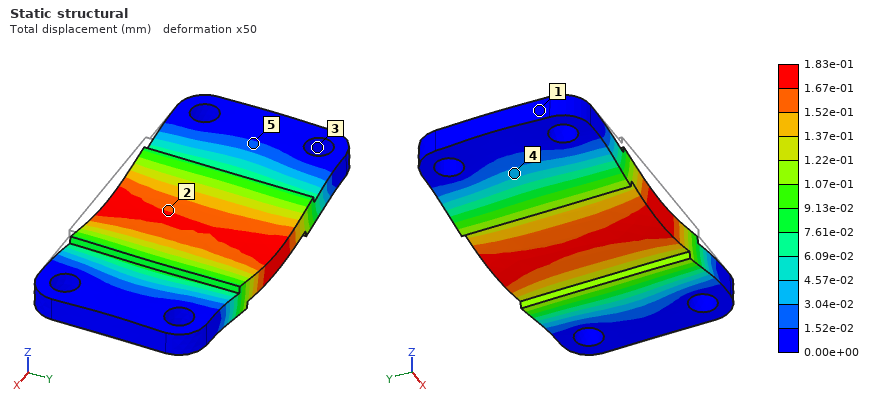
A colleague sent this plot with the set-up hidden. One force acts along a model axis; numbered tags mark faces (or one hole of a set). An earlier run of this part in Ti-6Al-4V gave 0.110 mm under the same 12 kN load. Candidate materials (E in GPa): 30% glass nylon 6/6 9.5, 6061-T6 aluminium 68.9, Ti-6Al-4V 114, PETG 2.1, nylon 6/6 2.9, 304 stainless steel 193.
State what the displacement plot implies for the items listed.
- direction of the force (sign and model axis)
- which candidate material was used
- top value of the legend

-Z
6061-T6 aluminium
1.83e-01 mm
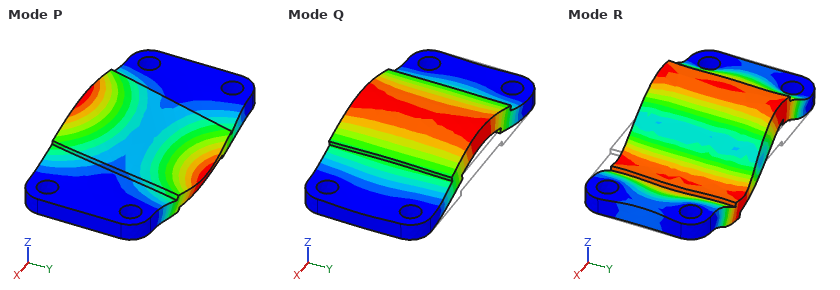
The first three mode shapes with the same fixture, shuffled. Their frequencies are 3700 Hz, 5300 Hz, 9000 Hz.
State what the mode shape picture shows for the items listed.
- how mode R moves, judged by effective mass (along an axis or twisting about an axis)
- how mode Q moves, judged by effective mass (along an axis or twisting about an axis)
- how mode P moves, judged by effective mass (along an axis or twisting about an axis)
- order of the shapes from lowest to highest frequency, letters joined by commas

twisting about Y
along Z
twisting about X
Q, P, R
